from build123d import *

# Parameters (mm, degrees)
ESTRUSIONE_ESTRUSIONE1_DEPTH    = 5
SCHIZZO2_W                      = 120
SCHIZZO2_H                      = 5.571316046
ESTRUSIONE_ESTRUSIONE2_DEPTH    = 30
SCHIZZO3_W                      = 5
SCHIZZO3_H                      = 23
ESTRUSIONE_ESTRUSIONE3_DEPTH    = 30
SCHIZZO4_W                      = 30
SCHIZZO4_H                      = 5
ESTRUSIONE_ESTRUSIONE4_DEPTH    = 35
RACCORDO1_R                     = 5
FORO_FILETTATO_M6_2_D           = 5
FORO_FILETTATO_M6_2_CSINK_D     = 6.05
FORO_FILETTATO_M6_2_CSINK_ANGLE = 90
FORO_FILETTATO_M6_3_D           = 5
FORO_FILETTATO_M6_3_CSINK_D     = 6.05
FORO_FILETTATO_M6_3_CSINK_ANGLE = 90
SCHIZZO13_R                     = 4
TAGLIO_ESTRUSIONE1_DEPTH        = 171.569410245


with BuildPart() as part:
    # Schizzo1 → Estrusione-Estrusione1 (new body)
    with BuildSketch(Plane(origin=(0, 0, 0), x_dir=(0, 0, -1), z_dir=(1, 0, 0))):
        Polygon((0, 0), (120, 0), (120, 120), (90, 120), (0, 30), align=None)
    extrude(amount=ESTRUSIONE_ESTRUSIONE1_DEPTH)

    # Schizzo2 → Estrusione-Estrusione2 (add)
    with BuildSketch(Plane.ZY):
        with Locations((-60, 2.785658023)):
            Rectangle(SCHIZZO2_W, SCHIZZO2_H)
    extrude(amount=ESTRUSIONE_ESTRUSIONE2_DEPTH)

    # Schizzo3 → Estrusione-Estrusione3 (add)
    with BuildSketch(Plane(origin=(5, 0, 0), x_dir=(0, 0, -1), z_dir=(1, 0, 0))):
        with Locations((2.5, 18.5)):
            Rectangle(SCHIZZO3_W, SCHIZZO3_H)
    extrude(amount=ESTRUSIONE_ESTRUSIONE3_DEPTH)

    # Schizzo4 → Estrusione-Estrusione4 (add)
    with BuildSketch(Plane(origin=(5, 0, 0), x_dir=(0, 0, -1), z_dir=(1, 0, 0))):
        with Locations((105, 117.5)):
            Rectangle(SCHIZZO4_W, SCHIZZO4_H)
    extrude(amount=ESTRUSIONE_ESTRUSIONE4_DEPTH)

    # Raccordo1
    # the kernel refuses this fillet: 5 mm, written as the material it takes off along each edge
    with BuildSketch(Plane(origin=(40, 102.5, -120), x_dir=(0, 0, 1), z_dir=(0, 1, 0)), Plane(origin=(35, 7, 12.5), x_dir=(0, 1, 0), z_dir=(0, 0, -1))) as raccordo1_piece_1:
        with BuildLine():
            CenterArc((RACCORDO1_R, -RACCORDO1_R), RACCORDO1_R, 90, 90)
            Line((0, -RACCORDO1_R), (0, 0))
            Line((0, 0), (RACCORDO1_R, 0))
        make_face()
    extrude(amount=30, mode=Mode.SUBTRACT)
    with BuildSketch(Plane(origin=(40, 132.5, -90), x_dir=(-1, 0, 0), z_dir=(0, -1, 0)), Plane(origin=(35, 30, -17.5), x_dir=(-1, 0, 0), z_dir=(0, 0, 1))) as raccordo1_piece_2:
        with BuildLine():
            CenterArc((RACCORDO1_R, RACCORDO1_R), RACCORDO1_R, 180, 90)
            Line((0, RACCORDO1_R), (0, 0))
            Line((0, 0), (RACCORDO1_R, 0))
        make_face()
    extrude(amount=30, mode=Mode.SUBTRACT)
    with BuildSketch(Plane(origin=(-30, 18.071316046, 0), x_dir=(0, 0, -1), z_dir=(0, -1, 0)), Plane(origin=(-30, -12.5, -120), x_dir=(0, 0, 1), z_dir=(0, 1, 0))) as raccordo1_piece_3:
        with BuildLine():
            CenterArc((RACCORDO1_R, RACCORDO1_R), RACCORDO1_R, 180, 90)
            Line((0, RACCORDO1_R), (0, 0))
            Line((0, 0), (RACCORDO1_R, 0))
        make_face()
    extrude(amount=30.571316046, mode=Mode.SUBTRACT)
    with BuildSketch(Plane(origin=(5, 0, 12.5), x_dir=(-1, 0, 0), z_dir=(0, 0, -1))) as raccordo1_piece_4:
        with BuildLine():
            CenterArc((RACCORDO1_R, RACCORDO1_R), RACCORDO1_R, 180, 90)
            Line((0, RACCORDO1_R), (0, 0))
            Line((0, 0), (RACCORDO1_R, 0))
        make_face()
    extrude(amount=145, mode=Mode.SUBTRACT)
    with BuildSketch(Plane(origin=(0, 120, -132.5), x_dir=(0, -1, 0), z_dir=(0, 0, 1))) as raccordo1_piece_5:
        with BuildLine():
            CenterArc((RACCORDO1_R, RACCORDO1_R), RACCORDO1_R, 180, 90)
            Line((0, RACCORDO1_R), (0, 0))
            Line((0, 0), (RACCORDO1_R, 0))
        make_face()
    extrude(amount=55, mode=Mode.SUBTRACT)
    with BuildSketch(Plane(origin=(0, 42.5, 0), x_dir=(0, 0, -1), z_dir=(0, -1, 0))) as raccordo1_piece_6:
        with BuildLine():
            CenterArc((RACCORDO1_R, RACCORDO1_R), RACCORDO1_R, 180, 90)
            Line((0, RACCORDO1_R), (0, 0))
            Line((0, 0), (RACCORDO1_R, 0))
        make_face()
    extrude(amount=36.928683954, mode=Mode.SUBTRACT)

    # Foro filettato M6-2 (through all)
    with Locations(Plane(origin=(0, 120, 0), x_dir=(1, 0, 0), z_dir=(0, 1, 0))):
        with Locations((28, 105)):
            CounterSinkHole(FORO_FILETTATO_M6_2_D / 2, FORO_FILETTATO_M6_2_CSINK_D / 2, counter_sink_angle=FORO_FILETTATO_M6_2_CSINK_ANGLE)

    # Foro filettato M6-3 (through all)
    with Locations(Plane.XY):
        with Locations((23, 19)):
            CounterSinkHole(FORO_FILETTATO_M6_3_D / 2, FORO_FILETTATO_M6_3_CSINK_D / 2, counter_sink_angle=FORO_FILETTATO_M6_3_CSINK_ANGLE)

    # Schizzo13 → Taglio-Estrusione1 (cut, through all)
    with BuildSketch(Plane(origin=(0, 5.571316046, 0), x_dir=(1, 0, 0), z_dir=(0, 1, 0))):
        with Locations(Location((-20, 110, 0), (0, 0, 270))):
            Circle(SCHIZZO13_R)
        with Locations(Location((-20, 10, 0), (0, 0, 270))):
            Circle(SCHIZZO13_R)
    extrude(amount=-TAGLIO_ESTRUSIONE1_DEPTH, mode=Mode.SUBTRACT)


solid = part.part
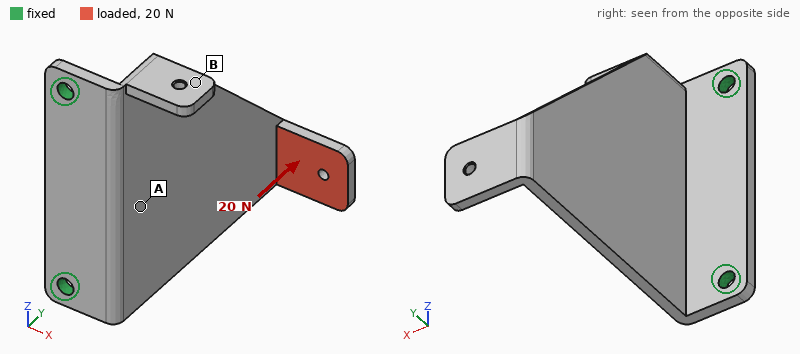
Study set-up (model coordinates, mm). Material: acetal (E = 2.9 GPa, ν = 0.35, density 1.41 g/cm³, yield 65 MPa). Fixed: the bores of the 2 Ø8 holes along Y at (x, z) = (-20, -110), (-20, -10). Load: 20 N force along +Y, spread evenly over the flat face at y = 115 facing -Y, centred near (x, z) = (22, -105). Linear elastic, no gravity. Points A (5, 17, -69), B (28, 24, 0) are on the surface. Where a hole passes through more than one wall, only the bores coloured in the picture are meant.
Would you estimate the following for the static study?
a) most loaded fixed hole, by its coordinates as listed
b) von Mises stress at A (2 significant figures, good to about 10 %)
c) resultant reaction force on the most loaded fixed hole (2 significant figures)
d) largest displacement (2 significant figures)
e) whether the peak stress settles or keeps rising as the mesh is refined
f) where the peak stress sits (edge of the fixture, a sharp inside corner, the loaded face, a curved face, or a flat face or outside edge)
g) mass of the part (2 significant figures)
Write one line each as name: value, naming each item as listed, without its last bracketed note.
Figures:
most loaded fixed hole, by its coordinates as listed: (-20, -110)
von Mises stress at A: 0.82 MPa
resultant reaction force on the most loaded fixed hole: 19 N
largest displacement: 2.0 mm
whether the peak stress settles or keeps rising as the mesh is refined: keeps rising
where the peak stress sits: edge of the fixture
mass of the part: 110 g
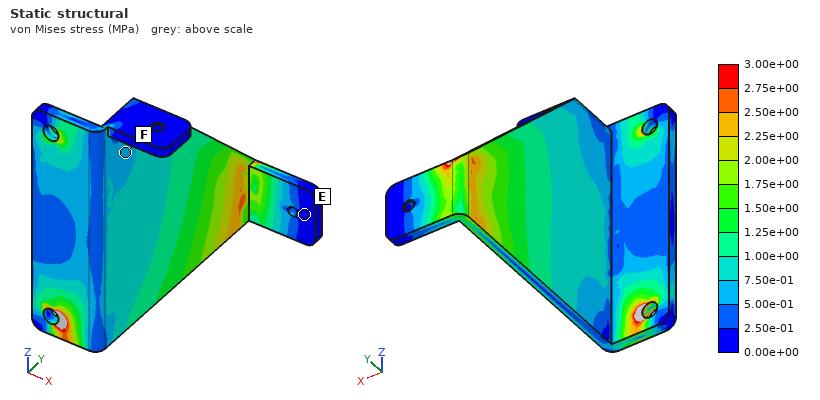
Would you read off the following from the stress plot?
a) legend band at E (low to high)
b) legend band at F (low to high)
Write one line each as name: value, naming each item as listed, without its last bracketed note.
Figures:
legend band at E: 0.00e+00 to 2.50e-01 MPa
legend band at F: 5.00e-01 to 7.50e-01 MPa
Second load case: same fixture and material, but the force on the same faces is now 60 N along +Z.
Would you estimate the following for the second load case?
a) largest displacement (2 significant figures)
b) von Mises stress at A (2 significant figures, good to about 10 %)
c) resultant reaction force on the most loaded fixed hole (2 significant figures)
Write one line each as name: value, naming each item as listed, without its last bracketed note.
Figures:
largest displacement: 2.2 mm
von Mises stress at A: 0.60 MPa
resultant reaction force on the most loaded fixed hole: 82 N
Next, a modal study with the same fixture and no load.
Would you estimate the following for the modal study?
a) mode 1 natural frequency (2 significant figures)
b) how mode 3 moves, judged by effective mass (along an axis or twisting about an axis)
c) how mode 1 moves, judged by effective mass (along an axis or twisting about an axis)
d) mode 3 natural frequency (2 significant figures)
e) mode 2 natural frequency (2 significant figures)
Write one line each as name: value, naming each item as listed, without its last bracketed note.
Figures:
mode 1 natural frequency: 71 Hz
how mode 3 moves, judged by effective mass: along Z
how mode 1 moves, judged by effective mass: along X
mode 3 natural frequency: 350 Hz
mode 2 natural frequency: 270 Hz
